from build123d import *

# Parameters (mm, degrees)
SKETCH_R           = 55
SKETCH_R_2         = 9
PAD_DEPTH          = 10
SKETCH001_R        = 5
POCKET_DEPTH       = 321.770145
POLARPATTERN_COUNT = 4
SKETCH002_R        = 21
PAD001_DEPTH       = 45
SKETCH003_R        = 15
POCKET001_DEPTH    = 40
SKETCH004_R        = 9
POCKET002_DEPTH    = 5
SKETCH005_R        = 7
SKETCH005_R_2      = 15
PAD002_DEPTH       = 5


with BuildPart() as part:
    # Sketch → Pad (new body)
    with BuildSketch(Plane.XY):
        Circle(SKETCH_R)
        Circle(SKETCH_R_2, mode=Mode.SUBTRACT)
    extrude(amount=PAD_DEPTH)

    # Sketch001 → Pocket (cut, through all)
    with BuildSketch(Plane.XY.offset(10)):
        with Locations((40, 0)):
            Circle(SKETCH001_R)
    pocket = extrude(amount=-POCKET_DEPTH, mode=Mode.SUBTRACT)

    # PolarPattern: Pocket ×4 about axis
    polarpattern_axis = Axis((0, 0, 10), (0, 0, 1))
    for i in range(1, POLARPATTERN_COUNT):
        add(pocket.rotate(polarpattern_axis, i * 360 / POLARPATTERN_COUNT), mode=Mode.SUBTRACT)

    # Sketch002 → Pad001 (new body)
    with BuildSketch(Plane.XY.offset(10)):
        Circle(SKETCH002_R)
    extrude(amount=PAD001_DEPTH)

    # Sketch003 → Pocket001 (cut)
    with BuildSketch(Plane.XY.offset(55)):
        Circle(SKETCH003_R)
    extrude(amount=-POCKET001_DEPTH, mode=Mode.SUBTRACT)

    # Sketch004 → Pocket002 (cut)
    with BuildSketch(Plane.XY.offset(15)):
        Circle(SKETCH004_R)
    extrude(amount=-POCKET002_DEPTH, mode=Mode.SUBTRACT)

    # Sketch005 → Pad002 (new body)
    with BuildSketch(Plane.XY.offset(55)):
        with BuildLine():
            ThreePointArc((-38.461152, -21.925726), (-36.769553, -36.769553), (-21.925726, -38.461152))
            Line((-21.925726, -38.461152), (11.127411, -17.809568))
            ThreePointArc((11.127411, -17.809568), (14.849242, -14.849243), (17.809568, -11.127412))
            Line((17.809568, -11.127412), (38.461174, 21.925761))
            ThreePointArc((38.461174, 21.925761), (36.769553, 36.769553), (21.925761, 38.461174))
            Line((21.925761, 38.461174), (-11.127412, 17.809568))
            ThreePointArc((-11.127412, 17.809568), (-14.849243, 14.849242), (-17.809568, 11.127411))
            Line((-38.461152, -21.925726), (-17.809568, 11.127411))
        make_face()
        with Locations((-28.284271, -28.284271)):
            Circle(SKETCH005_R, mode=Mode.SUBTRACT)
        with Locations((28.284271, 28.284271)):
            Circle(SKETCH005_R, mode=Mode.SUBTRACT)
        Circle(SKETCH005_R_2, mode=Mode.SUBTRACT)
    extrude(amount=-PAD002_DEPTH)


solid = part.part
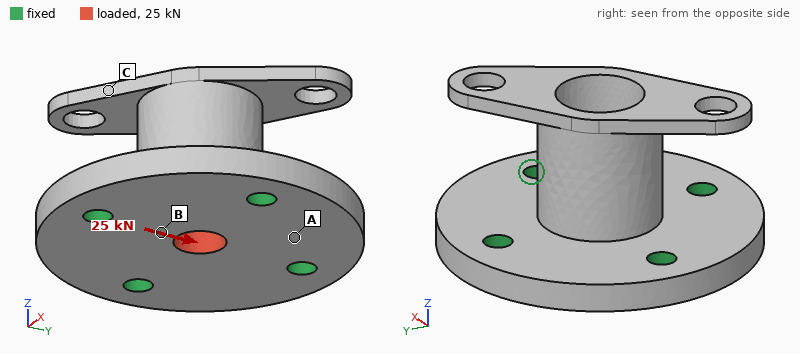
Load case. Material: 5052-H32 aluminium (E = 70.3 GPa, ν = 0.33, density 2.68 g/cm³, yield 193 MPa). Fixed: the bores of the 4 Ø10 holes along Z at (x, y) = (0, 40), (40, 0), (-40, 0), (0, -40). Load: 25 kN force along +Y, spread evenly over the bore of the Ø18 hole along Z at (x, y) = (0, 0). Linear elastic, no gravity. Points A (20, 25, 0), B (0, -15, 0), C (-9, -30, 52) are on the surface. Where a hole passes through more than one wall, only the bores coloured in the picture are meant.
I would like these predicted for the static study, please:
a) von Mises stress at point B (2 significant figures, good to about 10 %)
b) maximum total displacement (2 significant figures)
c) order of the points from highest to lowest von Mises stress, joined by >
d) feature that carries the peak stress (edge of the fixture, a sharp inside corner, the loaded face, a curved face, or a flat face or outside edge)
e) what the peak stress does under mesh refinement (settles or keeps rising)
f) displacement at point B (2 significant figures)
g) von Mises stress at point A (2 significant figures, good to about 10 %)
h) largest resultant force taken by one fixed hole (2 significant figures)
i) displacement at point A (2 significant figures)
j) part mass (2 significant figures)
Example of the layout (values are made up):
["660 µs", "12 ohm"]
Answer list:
["31 MPa", "17 µm", "B > A > C", "edge of the fixture", "keeps rising", "11 µm", "9.0 MPa", "8.3 kN", "7.3 µm", "350 g"]
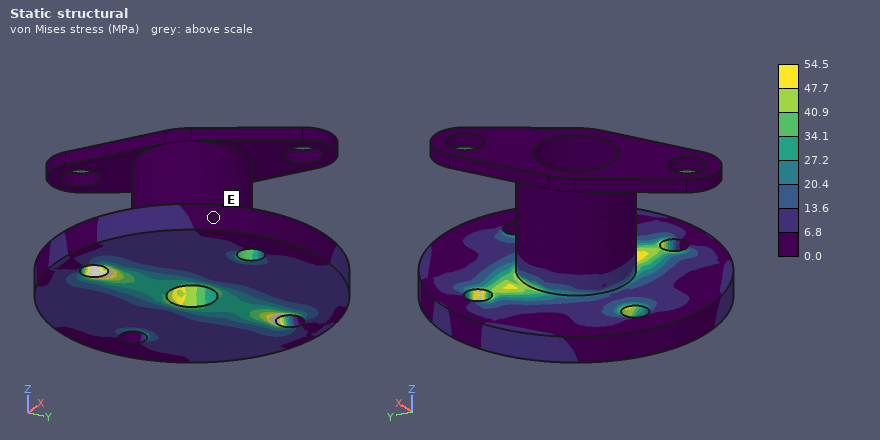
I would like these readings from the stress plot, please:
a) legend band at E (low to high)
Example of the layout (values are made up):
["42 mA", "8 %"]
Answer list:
["0.0 to 6.8 MPa"]
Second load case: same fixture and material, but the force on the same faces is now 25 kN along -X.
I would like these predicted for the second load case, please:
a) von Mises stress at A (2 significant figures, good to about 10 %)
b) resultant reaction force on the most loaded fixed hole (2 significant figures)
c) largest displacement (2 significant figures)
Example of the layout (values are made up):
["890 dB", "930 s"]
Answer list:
["8.3 MPa", "8.3 kN", "17 µm"]
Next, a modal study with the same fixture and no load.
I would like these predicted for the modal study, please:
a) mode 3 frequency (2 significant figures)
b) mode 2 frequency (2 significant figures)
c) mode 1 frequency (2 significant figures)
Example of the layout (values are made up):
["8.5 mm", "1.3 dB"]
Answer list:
["5300 Hz", "4500 Hz", "4100 Hz"]
